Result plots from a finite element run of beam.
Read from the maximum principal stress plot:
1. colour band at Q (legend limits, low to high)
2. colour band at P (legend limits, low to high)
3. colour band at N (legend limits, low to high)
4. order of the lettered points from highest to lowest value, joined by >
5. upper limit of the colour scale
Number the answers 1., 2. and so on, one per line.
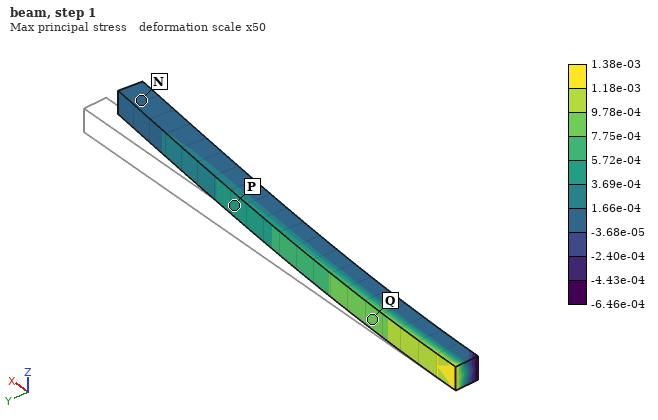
1. 7.75e-04 to 9.78e-04
2. 3.69e-04 to 5.72e-04
3. -3.68e-05 to 1.66e-04
4. Q > P > N
5. 1.38e-03
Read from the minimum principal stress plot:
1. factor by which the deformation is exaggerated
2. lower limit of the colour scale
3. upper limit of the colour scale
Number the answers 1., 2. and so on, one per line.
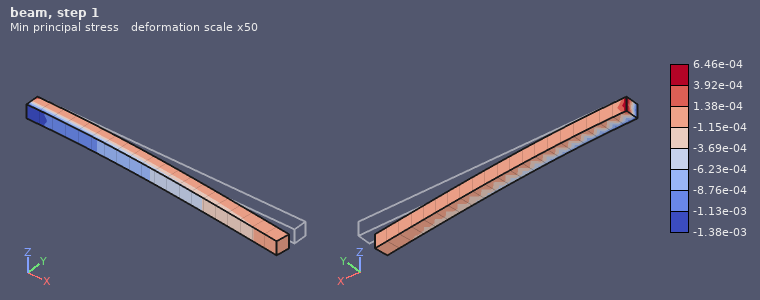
1. 50
2. -1.38e-03
3. 6.46e-04
